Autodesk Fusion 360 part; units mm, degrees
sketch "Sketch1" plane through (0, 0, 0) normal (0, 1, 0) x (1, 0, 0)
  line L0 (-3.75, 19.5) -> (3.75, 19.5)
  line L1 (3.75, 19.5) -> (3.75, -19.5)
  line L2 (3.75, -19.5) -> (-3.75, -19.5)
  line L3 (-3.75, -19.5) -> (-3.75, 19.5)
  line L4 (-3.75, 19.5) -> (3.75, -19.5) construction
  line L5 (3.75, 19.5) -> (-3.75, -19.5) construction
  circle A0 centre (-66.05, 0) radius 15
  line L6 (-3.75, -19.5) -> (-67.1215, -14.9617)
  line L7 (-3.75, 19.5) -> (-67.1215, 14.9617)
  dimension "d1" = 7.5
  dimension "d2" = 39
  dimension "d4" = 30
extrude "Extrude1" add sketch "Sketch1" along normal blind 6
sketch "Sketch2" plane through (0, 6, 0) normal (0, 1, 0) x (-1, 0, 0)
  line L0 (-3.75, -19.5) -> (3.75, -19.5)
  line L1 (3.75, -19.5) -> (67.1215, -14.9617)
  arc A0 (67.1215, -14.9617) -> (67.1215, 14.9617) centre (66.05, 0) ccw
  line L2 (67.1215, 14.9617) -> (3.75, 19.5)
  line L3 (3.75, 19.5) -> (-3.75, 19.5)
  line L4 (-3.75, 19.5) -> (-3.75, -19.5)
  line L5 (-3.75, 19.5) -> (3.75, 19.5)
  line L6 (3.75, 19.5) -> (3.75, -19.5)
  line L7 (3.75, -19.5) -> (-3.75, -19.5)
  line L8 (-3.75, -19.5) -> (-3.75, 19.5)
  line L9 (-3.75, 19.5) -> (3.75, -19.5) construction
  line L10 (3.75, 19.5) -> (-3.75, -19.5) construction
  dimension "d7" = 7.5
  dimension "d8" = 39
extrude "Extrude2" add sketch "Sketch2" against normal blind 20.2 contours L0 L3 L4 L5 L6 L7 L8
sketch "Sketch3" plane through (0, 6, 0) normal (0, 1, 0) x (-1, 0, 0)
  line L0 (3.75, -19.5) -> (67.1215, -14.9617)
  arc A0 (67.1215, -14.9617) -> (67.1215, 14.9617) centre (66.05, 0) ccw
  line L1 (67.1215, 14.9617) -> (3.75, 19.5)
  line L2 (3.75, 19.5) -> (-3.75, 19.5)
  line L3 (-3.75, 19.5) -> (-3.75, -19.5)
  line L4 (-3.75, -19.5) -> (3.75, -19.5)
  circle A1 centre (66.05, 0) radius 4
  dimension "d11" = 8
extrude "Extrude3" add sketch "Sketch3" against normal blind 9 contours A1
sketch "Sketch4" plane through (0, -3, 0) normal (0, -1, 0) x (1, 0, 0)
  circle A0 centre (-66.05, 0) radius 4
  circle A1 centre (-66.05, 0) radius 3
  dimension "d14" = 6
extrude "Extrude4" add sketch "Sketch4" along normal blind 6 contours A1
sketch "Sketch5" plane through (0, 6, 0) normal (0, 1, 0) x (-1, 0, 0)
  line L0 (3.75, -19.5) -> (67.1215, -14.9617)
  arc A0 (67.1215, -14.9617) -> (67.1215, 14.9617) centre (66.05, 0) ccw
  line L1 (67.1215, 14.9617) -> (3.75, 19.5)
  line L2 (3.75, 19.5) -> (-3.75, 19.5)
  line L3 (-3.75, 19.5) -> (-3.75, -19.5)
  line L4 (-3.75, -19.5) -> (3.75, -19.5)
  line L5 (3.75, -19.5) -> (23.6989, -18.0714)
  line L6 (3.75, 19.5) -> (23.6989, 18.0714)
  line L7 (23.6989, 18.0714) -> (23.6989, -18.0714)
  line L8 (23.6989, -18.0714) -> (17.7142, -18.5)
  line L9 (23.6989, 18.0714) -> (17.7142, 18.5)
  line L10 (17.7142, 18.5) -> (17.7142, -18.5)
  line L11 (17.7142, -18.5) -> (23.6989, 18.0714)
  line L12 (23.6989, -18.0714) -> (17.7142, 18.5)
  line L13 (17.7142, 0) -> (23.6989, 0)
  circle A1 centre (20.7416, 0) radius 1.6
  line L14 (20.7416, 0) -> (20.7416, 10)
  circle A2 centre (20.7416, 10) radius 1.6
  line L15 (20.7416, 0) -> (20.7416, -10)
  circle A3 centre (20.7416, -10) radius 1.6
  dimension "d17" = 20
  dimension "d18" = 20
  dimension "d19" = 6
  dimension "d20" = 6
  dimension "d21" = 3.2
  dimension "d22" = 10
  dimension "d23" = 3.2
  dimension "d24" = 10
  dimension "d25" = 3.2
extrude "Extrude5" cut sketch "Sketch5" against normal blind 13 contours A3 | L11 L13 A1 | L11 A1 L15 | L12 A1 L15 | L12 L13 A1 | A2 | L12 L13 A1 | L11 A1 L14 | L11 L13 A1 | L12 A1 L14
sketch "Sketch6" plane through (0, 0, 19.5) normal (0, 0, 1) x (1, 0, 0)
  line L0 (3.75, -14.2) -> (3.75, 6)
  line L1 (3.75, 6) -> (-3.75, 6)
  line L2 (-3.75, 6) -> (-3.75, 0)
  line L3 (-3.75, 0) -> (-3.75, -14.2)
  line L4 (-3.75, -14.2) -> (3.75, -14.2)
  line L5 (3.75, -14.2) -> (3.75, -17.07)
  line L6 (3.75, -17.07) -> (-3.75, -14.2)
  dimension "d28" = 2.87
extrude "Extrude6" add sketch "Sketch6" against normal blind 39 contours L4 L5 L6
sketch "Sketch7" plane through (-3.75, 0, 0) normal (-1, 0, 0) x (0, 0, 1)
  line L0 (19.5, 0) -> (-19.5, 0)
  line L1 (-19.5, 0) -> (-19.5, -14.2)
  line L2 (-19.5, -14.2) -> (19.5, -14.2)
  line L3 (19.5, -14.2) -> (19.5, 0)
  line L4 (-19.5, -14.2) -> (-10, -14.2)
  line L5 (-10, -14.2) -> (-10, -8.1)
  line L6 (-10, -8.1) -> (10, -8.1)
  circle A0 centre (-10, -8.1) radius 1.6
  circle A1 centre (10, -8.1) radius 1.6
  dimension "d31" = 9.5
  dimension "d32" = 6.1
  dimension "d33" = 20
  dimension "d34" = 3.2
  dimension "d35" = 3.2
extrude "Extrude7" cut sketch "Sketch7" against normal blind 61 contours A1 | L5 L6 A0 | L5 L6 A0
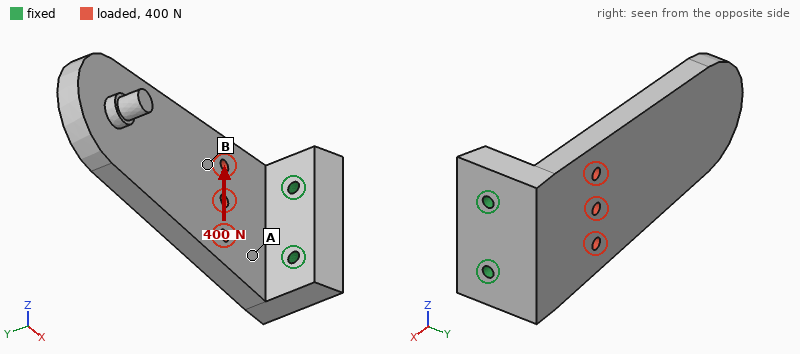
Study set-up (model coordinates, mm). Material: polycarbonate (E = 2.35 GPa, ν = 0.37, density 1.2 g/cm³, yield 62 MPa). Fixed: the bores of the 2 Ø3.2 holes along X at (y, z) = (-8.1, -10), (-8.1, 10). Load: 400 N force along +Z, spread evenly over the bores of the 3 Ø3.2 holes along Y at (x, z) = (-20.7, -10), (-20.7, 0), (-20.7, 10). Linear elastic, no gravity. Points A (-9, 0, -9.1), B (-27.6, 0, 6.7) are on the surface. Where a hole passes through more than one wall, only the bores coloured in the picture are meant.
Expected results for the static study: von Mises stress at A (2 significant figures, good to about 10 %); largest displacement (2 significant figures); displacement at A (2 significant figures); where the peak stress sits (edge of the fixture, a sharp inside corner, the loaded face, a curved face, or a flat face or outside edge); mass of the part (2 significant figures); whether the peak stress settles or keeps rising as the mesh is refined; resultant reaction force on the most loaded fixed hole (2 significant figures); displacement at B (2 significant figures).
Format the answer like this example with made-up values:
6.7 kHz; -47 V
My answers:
7.2 MPa; 0.84 mm; 0.15 mm; edge of the fixture; 26 g; keeps rising; 430 N; 0.35 mm
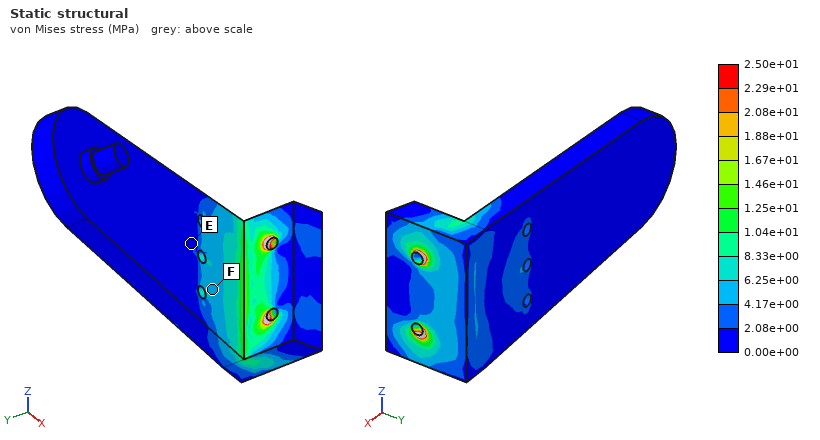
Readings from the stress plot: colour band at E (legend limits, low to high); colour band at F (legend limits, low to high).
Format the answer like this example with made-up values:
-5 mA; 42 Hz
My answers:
0.00e+00 to 2.08e+00 MPa; 4.17e+00 to 6.25e+00 MPa
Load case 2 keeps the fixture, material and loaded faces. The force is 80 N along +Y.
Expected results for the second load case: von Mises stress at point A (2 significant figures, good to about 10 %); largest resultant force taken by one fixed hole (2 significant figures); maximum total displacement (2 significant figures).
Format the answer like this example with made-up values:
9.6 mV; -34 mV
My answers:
3.8 MPa; 42 N; 1.1 mm
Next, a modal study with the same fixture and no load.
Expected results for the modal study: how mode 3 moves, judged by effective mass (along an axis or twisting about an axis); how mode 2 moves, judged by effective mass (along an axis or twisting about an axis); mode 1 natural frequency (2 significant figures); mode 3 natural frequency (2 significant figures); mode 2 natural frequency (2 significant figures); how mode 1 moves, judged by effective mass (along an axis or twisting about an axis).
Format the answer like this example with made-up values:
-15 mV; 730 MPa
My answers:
twisting about X; along Z; 210 Hz; 1200 Hz; 670 Hz; along Y
